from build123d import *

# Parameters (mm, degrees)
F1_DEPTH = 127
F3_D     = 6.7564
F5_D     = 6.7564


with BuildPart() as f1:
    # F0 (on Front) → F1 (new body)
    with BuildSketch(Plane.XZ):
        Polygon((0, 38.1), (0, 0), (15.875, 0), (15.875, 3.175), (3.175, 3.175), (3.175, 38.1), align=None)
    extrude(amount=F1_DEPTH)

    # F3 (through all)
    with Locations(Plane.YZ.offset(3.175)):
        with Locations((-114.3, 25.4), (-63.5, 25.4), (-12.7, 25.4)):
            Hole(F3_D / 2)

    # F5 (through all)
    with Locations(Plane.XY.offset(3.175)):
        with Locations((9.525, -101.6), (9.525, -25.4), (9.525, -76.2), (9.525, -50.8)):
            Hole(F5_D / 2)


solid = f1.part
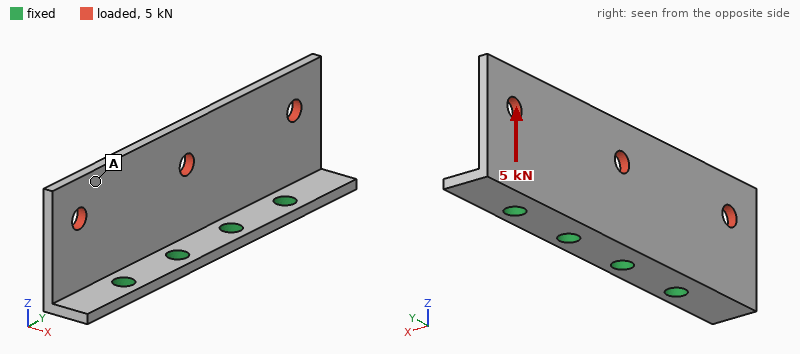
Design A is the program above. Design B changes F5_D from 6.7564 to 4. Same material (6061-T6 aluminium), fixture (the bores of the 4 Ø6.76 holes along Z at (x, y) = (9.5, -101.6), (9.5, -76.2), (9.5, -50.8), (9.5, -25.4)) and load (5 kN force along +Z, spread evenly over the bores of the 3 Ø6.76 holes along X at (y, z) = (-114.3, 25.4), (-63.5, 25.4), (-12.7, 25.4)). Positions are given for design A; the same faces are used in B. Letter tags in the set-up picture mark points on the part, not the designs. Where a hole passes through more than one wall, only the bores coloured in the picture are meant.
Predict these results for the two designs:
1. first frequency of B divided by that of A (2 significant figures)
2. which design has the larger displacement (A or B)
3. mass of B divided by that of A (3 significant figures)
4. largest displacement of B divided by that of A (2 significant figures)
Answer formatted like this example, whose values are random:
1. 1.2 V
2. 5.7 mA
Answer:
1. 0.92
2. B
3. 1.02
4. 1.6
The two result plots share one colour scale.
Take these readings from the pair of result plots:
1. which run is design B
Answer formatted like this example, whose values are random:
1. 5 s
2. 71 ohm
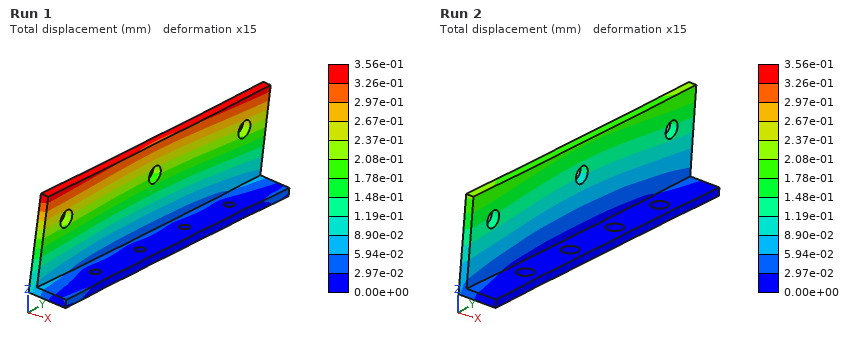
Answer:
1. Run 1
